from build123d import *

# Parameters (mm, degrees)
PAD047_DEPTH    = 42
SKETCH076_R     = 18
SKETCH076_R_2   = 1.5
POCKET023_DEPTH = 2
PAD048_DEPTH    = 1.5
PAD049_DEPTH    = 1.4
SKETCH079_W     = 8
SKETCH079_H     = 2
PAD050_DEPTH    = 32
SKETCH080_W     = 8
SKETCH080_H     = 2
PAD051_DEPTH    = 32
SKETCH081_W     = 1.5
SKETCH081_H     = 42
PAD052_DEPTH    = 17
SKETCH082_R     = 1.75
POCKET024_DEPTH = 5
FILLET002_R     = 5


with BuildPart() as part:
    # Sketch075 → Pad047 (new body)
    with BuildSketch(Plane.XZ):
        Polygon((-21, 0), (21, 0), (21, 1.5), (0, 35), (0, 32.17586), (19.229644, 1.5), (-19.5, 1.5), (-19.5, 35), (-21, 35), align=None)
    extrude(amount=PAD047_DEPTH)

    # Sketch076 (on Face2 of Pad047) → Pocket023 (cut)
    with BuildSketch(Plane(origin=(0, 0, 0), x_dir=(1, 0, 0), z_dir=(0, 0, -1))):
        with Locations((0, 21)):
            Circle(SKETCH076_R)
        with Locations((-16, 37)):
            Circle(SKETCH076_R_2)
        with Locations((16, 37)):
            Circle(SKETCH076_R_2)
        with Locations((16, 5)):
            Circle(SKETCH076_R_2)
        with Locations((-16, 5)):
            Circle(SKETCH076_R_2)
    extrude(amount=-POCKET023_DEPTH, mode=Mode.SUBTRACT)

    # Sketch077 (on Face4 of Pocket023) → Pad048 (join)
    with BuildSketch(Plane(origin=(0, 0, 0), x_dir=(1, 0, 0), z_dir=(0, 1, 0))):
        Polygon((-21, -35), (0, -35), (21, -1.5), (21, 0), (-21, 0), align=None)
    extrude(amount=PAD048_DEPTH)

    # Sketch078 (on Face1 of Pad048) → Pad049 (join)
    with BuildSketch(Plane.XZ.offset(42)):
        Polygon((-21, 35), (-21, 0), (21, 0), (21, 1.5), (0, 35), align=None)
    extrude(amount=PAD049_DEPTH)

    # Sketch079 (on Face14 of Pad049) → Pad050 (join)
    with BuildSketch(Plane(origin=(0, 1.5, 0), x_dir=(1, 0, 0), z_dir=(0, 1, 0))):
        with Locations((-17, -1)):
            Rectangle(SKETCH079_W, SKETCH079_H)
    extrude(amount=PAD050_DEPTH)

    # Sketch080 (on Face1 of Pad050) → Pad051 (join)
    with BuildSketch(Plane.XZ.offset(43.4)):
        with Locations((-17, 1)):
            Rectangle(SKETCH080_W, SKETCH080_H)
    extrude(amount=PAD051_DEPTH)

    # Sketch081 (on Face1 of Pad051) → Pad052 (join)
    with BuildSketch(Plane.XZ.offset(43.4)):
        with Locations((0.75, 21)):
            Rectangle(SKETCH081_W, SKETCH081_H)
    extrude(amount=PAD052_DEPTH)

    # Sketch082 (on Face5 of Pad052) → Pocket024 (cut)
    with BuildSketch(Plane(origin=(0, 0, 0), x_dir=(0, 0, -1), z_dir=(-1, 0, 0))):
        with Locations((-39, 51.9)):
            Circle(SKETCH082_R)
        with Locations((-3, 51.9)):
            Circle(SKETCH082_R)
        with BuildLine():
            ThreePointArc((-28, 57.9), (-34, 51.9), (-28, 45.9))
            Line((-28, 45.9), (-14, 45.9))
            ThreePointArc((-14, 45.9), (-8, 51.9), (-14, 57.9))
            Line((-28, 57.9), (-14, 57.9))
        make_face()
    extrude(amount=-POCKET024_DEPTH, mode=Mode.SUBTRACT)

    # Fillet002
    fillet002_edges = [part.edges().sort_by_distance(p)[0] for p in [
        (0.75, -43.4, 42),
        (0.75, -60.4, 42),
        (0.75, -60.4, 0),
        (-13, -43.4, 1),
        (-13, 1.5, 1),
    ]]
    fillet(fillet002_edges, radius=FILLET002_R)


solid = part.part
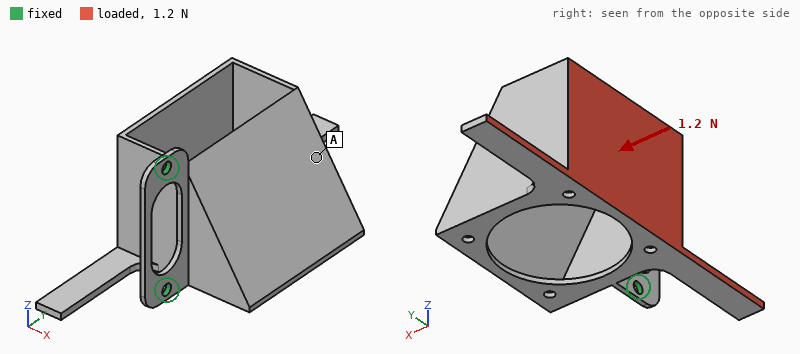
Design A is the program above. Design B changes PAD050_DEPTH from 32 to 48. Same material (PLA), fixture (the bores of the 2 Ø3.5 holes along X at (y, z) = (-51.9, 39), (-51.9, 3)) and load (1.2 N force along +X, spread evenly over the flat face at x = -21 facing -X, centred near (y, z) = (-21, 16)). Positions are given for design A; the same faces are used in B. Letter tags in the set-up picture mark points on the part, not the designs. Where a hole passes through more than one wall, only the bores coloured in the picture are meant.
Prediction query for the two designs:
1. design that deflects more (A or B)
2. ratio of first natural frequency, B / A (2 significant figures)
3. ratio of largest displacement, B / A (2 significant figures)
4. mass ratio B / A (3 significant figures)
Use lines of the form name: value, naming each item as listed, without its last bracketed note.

design that deflects more: B
ratio of first natural frequency, B / A: 0.92
ratio of largest displacement, B / A: 1.2
mass ratio B / A: 1.02
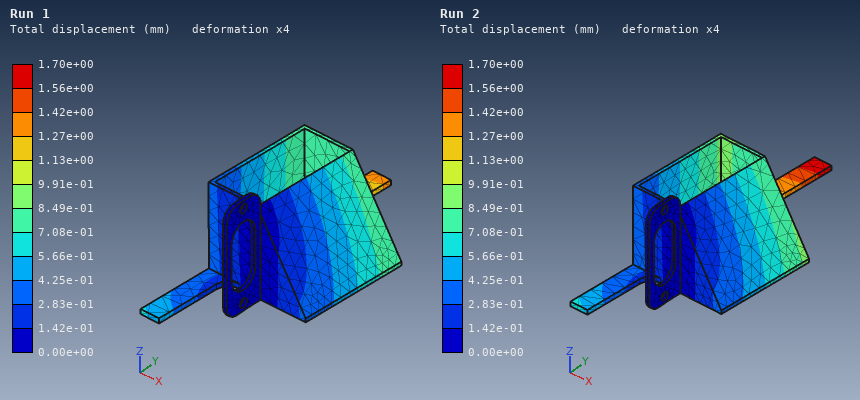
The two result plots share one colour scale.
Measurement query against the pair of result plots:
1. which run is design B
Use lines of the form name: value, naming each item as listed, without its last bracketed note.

which run is design B: Run 2
